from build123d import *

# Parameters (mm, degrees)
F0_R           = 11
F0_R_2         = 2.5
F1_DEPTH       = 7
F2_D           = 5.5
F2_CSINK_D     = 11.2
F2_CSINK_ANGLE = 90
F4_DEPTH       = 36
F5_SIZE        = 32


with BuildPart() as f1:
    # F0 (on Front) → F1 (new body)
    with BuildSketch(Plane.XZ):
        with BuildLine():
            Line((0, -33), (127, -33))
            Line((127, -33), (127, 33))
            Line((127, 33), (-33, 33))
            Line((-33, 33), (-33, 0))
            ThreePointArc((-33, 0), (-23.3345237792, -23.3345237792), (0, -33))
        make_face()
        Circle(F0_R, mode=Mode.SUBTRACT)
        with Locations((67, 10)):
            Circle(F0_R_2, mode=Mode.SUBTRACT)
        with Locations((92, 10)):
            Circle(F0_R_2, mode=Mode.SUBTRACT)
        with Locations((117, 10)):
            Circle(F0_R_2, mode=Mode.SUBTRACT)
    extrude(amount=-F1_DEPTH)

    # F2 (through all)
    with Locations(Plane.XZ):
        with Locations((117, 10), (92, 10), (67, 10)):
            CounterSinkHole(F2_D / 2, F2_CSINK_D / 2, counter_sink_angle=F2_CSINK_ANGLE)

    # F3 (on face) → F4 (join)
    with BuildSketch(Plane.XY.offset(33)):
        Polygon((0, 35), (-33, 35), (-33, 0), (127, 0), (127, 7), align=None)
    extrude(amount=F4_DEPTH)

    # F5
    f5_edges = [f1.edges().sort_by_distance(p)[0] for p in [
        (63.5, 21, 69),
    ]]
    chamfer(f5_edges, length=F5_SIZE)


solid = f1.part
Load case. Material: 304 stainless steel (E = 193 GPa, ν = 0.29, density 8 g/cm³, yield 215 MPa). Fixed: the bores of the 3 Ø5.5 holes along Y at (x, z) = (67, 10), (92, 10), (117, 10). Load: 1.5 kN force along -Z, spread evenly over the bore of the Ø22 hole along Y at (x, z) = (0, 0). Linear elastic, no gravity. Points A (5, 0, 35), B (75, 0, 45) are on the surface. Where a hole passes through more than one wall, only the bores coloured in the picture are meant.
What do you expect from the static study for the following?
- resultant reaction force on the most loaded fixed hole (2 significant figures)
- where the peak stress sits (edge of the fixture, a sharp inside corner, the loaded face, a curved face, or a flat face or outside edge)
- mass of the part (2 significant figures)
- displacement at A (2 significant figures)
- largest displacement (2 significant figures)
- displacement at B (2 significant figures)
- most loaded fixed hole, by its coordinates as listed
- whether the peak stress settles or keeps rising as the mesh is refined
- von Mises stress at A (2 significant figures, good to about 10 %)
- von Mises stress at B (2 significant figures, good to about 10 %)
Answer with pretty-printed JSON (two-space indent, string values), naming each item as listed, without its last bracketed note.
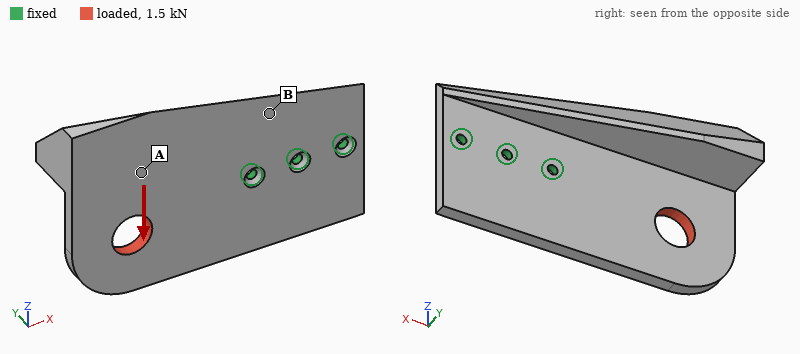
{
  "resultant reaction force on the most loaded fixed hole": "3.4 kN",
  "where the peak stress sits": "edge of the fixture",
  "mass of the part": "1.1 kg",
  "displacement at A": "13 µm",
  "largest displacement": "21 µm",
  "displacement at B": "4.4 µm",
  "most loaded fixed hole, by its coordinates as listed": "(67, 10)",
  "whether the peak stress settles or keeps rising as the mesh is refined": "keeps rising",
  "von Mises stress at A": "3.5 MPa",
  "von Mises stress at B": "9.8 MPa"
}
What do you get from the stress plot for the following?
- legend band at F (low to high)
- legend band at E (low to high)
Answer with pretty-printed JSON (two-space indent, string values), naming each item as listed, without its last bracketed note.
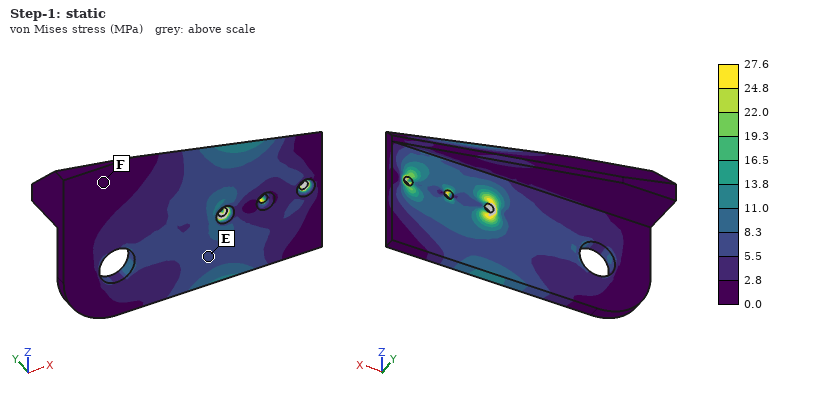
{
  "legend band at F": "0.0 to 2.8 MPa",
  "legend band at E": "5.5 to 8.3 MPa"
}
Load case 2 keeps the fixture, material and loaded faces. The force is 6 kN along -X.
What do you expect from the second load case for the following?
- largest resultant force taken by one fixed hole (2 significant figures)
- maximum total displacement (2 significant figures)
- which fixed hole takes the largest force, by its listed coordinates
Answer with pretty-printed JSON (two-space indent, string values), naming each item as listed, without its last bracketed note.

{
  "largest resultant force taken by one fixed hole": "3.6 kN",
  "maximum total displacement": "17 µm",
  "which fixed hole takes the largest force, by its listed coordinates": "(67, 10)"
}
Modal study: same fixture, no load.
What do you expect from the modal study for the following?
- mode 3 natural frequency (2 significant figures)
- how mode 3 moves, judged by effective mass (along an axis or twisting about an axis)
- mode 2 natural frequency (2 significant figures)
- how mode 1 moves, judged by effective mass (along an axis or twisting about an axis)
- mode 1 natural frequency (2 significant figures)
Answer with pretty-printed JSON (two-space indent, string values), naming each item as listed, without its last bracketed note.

{
  "mode 3 natural frequency": "1900 Hz",
  "how mode 3 moves, judged by effective mass": "along Z",
  "mode 2 natural frequency": "940 Hz",
  "how mode 1 moves, judged by effective mass": "along Y",
  "mode 1 natural frequency": "450 Hz"
}
